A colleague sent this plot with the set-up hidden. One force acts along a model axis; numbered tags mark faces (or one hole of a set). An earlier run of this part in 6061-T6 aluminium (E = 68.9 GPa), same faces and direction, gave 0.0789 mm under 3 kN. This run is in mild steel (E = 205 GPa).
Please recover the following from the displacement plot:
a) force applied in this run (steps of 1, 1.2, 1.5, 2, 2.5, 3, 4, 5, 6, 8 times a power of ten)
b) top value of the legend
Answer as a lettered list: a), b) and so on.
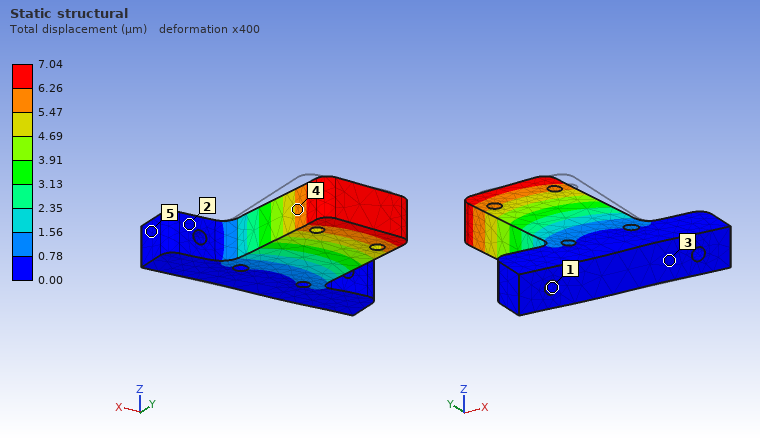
a) 800 N
b) 7.04 µm
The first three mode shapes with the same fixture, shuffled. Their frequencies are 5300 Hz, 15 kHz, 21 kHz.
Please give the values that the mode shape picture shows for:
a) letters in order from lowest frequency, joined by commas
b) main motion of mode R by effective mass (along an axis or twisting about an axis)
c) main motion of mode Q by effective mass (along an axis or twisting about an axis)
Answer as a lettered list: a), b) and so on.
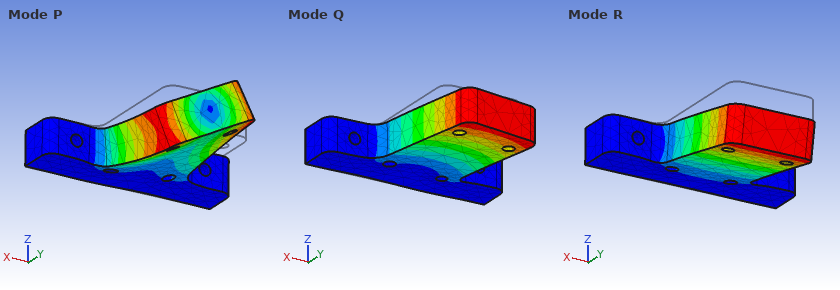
a) R, Q, P
b) along Z
c) along X
